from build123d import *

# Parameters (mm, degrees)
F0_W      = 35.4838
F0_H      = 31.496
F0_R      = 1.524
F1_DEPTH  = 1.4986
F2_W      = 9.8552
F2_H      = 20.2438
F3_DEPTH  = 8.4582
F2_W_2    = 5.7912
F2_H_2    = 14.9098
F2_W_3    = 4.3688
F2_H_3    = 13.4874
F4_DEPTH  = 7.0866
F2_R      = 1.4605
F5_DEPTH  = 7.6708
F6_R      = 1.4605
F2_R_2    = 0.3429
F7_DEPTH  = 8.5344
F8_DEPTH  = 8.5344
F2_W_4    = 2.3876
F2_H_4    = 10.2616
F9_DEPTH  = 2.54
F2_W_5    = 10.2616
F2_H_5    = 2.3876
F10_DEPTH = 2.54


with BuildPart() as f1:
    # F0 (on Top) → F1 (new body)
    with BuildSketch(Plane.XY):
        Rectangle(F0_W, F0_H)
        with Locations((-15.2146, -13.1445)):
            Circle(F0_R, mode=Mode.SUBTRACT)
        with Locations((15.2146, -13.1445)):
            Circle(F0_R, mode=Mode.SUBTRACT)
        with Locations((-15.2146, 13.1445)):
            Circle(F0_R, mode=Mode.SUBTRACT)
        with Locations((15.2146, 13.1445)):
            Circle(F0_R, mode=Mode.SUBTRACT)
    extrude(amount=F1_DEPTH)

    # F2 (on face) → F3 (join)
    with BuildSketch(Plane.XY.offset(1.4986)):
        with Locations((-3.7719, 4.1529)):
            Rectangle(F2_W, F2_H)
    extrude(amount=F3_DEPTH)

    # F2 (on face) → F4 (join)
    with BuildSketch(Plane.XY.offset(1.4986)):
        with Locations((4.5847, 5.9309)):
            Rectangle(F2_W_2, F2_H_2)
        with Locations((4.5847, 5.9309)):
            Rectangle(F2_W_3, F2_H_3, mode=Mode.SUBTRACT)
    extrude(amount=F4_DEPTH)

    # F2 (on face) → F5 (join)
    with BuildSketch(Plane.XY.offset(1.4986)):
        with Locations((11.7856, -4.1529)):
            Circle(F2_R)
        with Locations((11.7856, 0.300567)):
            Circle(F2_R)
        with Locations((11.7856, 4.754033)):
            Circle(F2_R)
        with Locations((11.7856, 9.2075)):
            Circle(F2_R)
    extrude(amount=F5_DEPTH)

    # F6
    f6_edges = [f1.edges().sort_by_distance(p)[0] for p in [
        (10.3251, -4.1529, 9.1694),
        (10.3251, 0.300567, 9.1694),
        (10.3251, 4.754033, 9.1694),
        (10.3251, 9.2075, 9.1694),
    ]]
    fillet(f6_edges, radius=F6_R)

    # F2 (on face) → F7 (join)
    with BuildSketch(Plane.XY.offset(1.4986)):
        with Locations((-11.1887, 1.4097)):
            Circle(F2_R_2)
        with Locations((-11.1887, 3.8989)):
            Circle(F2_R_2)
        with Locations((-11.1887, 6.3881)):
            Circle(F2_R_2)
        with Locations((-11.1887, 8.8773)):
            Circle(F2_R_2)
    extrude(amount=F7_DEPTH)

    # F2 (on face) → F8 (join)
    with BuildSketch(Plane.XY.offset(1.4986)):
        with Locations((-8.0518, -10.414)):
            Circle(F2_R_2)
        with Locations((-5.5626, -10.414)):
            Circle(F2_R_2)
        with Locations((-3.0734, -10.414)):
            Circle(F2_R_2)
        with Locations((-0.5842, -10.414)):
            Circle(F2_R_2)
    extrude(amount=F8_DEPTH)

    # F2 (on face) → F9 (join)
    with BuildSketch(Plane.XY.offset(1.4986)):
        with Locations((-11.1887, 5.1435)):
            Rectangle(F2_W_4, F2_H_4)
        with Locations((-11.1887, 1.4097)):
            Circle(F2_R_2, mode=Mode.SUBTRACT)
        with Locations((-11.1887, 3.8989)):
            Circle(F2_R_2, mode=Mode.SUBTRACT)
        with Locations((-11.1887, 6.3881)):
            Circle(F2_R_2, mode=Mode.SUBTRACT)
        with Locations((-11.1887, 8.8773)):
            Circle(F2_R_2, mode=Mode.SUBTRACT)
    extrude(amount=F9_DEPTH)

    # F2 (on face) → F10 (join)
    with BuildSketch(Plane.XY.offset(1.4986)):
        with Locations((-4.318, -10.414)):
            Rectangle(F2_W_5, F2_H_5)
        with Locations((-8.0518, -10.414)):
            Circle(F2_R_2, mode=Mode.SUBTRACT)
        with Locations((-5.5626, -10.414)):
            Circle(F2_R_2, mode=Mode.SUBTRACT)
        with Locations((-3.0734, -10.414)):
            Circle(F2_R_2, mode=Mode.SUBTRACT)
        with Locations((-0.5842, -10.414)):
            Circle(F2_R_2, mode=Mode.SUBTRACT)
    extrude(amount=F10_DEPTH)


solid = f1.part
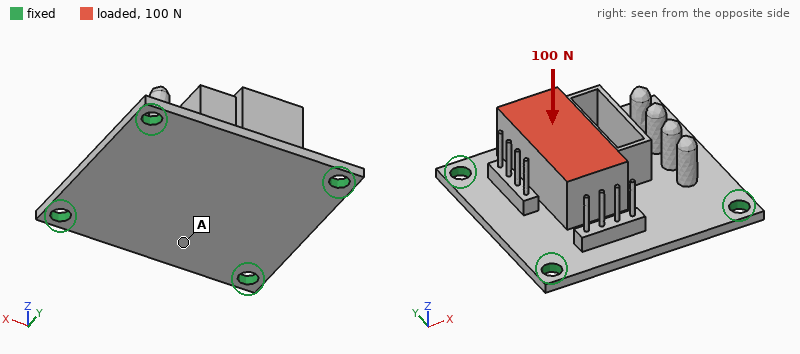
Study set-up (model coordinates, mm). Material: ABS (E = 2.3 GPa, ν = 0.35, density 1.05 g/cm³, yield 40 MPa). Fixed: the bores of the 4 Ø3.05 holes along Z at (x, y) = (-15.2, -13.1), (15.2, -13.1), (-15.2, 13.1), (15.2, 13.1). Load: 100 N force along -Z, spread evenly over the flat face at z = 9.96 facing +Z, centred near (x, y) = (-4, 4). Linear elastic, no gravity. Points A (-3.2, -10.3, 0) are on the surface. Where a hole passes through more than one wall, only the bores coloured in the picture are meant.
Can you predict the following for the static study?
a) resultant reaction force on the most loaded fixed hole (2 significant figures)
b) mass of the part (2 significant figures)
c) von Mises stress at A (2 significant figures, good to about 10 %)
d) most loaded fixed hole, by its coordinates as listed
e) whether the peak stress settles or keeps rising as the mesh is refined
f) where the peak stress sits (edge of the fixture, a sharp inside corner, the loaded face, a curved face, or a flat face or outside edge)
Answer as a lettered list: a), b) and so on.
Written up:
a) 48 N
b) 4.0 g
c) 4.4 MPa
d) (-15.2, 13.1)
e) keeps rising
f) edge of the fixture
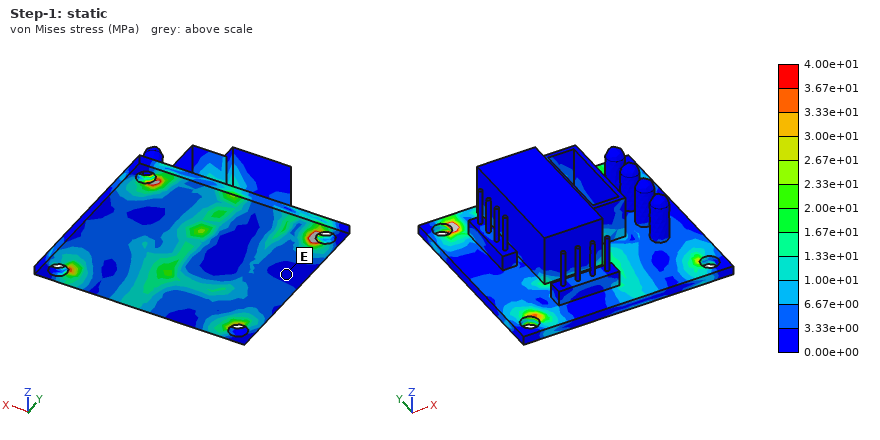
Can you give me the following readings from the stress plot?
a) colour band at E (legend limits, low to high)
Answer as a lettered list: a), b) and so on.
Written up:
a) 0.00e+00 to 3.33e+00 MPa
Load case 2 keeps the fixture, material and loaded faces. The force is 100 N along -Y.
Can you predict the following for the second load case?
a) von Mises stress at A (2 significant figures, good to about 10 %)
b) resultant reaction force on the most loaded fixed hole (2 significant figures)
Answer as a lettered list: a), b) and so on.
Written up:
a) 6.3 MPa
b) 54 N
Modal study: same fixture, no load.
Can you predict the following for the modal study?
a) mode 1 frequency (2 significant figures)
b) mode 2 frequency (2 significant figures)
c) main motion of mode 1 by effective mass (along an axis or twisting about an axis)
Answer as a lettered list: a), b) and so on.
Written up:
a) 1400 Hz
b) 2300 Hz
c) along Z
